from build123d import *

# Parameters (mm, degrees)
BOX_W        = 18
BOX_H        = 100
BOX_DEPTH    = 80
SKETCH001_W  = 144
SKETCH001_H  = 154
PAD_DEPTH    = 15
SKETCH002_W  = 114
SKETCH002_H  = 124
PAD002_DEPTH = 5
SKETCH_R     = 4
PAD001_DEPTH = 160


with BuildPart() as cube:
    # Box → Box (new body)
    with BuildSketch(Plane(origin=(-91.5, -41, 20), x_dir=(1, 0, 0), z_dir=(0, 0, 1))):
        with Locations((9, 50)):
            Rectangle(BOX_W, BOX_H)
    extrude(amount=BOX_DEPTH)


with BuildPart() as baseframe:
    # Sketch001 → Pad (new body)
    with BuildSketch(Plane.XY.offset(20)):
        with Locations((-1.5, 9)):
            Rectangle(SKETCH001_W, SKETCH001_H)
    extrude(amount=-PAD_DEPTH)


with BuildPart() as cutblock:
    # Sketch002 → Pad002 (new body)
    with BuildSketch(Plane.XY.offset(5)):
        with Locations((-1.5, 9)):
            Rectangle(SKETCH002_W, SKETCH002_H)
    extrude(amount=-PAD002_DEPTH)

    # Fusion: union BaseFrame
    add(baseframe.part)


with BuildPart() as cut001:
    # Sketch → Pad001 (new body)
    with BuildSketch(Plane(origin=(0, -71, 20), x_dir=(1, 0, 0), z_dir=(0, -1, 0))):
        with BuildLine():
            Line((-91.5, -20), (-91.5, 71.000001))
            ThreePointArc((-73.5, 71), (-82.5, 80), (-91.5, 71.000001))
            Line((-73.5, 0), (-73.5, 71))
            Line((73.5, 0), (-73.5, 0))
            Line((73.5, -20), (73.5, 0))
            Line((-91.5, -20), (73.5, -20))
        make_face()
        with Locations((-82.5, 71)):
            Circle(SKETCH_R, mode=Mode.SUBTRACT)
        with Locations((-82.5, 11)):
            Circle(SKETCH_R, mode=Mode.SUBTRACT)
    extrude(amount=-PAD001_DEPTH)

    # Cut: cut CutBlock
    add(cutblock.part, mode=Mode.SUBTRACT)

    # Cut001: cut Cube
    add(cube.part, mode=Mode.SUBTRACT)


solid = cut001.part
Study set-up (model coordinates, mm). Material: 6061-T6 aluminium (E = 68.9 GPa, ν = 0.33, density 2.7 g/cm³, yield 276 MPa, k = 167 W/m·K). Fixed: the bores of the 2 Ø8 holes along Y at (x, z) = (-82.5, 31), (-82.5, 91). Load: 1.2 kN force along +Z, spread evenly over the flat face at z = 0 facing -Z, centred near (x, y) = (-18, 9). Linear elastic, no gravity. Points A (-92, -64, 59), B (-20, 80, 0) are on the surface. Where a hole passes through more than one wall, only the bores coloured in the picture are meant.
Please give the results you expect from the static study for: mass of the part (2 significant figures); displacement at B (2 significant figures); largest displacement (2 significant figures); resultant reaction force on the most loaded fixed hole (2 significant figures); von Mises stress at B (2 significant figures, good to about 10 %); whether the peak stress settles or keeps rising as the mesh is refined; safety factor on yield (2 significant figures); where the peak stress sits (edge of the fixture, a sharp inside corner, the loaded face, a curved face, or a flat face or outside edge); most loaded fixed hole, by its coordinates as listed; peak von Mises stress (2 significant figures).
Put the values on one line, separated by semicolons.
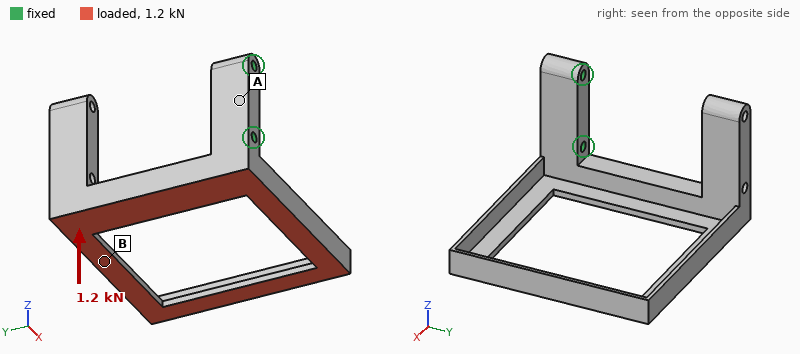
550 g; 1.2 mm; 2.8 mm; 1.2 kN; 21 MPa; settles; 1.9; a flat face or outside edge; (-82.5, 31); 150 MPa
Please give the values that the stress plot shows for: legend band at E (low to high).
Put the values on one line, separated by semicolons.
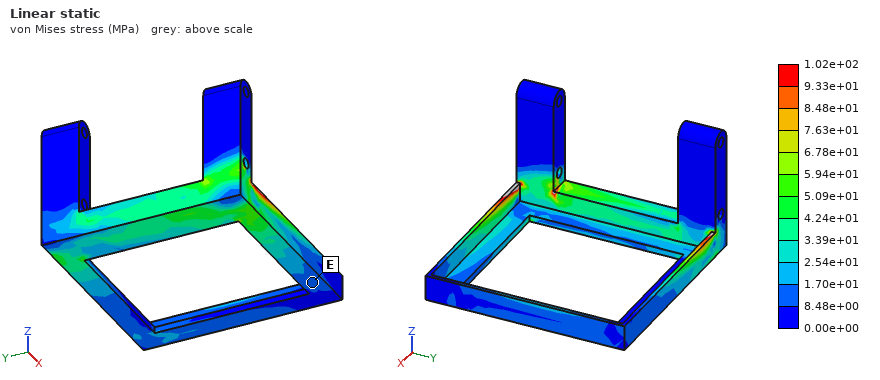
8.48e+00 to 1.70e+01 MPa
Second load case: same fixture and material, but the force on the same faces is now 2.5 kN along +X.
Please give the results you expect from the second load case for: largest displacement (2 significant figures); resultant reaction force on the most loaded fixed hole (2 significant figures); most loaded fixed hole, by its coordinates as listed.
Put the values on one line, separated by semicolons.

1.5 mm; 2.8 kN; (-82.5, 31)
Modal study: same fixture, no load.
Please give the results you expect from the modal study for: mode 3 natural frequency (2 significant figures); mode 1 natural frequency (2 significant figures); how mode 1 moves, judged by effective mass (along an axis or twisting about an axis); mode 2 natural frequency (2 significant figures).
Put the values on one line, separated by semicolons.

430 Hz; 240 Hz; along Z; 300 Hz
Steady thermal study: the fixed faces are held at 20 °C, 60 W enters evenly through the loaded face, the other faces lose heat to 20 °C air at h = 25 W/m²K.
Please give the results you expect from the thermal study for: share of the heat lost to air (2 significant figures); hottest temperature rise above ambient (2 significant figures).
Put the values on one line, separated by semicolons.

50 %; 43 K
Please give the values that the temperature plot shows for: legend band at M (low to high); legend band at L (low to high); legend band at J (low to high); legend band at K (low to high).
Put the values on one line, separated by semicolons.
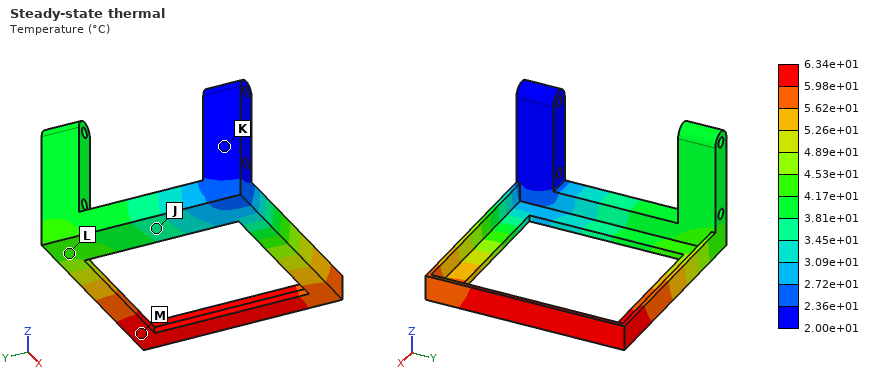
5.98e+01 to 6.34e+01 °C; 4.17e+01 to 4.53e+01 °C; 3.45e+01 to 3.81e+01 °C; 2.00e+01 to 2.36e+01 °C
